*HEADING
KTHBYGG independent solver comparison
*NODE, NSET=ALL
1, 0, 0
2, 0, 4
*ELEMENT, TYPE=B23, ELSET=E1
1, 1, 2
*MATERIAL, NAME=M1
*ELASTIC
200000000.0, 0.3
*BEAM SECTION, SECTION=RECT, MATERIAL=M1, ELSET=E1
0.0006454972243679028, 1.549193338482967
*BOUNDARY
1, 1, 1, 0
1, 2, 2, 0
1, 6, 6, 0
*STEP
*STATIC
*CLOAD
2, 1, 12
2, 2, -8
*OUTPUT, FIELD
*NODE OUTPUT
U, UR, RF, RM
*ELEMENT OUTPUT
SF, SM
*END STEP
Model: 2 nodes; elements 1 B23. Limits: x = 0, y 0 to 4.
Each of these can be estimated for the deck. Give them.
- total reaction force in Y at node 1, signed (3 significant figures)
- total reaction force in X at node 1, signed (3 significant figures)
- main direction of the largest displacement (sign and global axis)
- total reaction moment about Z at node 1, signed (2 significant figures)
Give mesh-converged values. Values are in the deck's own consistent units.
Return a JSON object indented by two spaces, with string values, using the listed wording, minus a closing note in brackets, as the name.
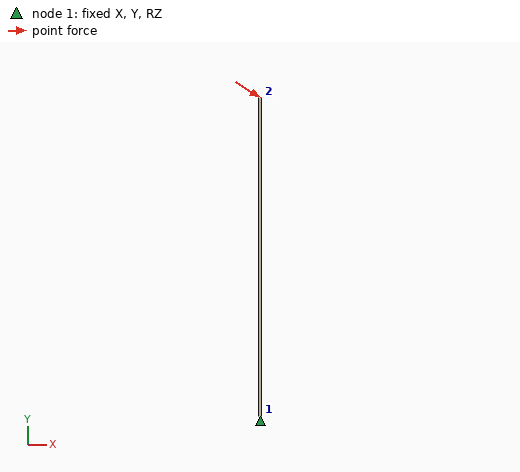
{
  "total reaction force in Y at node 1, signed": "8.00",
  "total reaction force in X at node 1, signed": "-12.0",
  "main direction of the largest displacement": "+X",
  "total reaction moment about Z at node 1, signed": "48"
}
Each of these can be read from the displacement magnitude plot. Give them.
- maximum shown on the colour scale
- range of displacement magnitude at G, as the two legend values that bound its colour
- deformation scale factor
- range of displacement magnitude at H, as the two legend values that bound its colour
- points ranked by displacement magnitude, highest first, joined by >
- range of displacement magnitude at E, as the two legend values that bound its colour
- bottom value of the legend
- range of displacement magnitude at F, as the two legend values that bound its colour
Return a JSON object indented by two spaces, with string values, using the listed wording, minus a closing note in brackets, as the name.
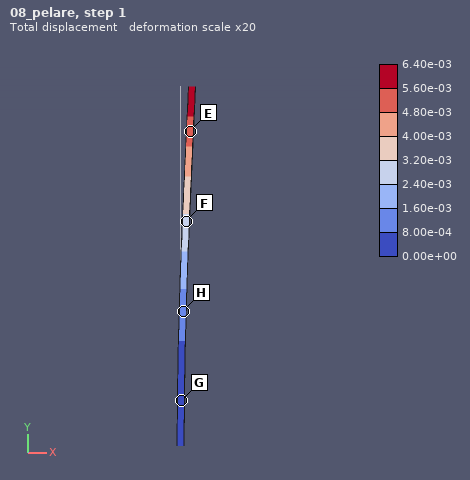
{
  "maximum shown on the colour scale": "6.40e-03",
  "range of displacement magnitude at G, as the two legend values that bound its colour": "0.00e+00 to 8.00e-04",
  "deformation scale factor": "20",
  "range of displacement magnitude at H, as the two legend values that bound its colour": "8.00e-04 to 1.60e-03",
  "points ranked by displacement magnitude, highest first, joined by >": "E > F > H > G",
  "range of displacement magnitude at E, as the two legend values that bound its colour": "4.80e-03 to 5.60e-03",
  "bottom value of the legend": "0.00e+00",
  "range of displacement magnitude at F, as the two legend values that bound its colour": "2.40e-03 to 3.20e-03"
}
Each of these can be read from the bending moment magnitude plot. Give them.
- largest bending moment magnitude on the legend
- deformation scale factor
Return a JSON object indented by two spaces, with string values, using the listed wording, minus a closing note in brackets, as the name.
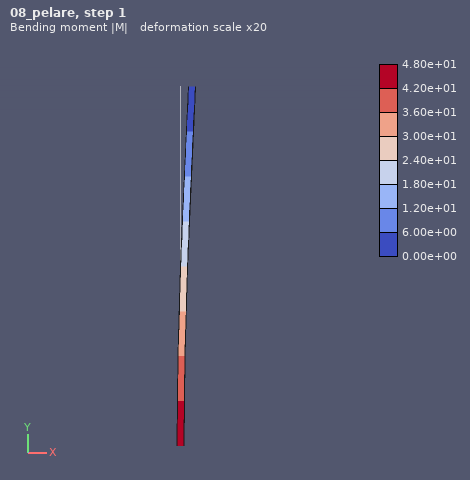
{
  "largest bending moment magnitude on the legend": "4.80e+01",
  "deformation scale factor": "20"
}
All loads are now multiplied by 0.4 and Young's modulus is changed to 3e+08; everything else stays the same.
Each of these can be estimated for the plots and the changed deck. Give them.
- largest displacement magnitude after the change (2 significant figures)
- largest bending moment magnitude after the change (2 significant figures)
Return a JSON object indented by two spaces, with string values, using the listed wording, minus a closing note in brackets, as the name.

{
  "largest displacement magnitude after the change": "0.0017",
  "largest bending moment magnitude after the change": "19"
}
